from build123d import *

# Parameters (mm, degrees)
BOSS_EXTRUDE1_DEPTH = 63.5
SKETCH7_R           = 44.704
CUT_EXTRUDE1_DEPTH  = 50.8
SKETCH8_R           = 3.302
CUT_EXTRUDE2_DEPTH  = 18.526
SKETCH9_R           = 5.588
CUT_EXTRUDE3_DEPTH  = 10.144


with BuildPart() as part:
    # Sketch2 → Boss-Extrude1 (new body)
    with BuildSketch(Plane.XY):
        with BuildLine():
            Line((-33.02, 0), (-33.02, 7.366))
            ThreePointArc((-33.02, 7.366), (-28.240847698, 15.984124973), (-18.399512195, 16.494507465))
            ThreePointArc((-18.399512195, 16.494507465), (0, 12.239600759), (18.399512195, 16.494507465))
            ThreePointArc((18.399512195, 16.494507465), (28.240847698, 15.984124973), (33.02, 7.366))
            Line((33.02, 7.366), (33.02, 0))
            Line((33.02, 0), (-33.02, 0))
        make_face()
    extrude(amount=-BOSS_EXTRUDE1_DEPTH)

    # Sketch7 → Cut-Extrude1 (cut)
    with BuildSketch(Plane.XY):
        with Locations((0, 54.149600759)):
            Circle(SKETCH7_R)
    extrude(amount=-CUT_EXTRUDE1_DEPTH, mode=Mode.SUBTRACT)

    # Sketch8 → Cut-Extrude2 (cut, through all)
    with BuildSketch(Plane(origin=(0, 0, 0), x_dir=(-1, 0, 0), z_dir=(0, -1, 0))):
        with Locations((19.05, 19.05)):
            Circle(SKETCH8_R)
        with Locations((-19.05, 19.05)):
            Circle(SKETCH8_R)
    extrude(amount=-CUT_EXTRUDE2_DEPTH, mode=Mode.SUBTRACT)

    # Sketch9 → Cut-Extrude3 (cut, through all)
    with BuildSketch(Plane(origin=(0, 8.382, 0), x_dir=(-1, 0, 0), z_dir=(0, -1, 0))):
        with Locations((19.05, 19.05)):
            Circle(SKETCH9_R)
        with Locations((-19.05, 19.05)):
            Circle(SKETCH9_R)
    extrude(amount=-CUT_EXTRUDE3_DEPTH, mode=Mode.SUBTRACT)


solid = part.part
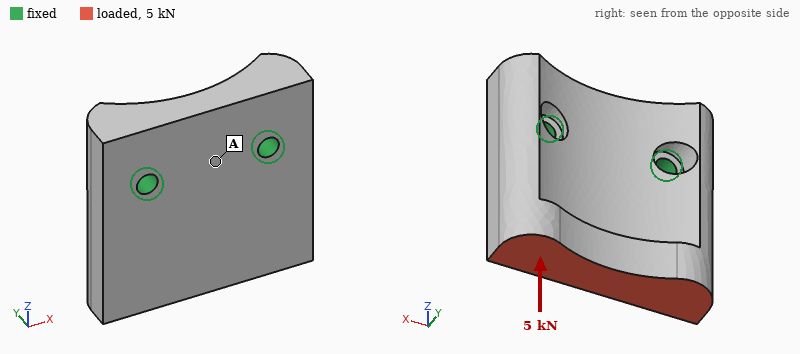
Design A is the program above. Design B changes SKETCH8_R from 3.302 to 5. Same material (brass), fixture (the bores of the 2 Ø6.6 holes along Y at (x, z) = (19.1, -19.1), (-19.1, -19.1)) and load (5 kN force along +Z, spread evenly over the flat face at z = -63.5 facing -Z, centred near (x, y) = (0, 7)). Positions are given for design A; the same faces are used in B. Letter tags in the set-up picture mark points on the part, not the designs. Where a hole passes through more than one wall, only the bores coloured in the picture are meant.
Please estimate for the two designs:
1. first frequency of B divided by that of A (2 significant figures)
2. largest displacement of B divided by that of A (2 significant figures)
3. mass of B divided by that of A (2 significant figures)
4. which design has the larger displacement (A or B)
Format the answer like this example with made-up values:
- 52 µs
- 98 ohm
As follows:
- 1.2
- 0.67
- 0.99
- A
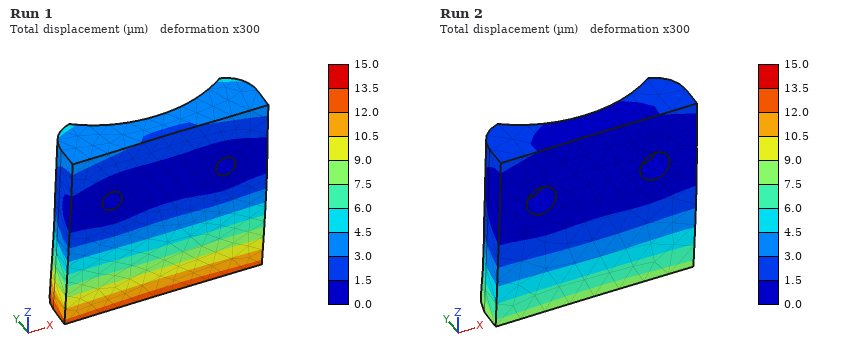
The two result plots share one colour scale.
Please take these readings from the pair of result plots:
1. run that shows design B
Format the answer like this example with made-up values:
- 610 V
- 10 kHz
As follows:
- Run 2
